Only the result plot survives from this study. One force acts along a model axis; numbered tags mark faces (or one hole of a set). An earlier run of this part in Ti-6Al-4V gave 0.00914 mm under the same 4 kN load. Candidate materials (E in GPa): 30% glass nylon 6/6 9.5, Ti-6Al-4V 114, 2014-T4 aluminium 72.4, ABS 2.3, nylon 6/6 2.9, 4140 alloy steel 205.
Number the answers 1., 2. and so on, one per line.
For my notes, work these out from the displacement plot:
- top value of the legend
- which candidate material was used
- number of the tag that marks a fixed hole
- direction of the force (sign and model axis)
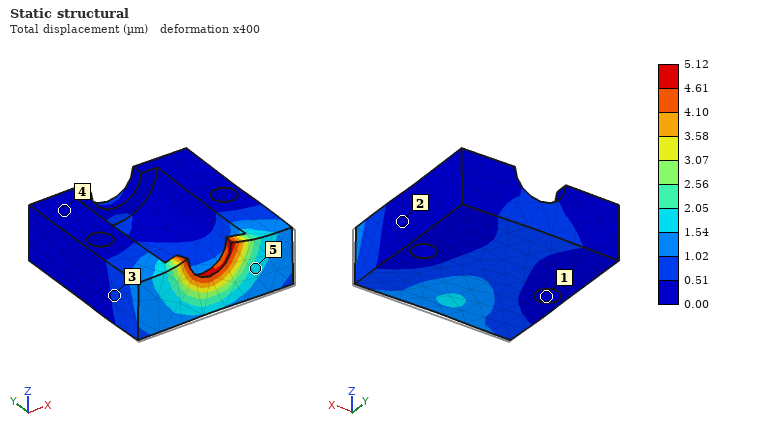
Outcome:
1. 5.12 µm
2. 4140 alloy steel
3. 1
4. +Y
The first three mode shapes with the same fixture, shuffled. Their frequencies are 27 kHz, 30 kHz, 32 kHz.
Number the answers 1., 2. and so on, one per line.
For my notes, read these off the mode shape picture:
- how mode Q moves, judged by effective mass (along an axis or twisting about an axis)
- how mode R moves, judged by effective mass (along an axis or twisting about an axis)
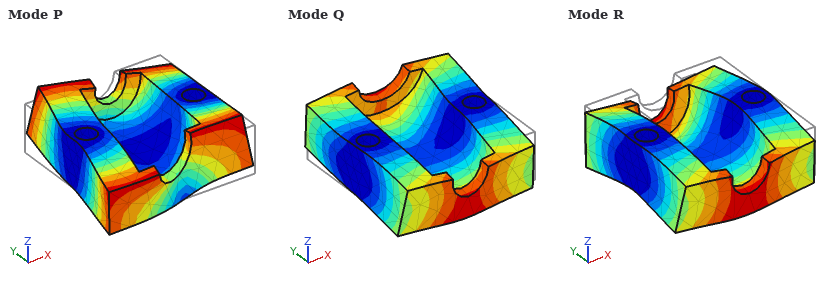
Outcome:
1. twisting about X
2. along Z
